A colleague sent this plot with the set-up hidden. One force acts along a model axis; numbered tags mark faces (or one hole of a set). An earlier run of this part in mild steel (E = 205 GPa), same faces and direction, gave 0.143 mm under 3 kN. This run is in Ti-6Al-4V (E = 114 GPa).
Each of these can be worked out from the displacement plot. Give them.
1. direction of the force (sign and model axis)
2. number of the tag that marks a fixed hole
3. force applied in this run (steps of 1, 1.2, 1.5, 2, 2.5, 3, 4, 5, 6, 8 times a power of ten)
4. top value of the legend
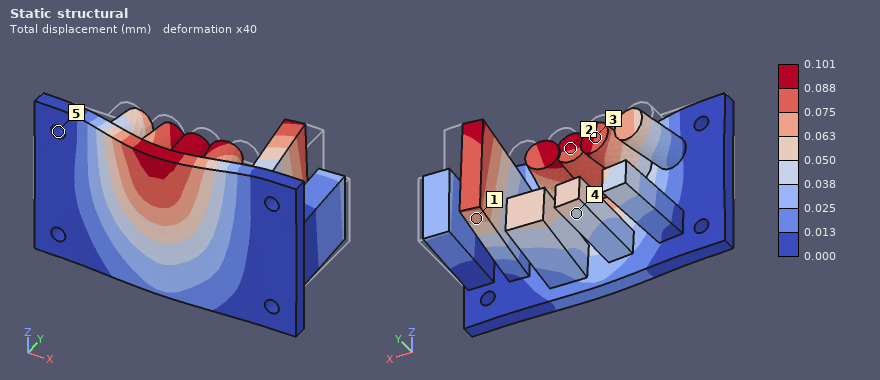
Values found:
-Y
5
1.2 kN
0.101 mm
